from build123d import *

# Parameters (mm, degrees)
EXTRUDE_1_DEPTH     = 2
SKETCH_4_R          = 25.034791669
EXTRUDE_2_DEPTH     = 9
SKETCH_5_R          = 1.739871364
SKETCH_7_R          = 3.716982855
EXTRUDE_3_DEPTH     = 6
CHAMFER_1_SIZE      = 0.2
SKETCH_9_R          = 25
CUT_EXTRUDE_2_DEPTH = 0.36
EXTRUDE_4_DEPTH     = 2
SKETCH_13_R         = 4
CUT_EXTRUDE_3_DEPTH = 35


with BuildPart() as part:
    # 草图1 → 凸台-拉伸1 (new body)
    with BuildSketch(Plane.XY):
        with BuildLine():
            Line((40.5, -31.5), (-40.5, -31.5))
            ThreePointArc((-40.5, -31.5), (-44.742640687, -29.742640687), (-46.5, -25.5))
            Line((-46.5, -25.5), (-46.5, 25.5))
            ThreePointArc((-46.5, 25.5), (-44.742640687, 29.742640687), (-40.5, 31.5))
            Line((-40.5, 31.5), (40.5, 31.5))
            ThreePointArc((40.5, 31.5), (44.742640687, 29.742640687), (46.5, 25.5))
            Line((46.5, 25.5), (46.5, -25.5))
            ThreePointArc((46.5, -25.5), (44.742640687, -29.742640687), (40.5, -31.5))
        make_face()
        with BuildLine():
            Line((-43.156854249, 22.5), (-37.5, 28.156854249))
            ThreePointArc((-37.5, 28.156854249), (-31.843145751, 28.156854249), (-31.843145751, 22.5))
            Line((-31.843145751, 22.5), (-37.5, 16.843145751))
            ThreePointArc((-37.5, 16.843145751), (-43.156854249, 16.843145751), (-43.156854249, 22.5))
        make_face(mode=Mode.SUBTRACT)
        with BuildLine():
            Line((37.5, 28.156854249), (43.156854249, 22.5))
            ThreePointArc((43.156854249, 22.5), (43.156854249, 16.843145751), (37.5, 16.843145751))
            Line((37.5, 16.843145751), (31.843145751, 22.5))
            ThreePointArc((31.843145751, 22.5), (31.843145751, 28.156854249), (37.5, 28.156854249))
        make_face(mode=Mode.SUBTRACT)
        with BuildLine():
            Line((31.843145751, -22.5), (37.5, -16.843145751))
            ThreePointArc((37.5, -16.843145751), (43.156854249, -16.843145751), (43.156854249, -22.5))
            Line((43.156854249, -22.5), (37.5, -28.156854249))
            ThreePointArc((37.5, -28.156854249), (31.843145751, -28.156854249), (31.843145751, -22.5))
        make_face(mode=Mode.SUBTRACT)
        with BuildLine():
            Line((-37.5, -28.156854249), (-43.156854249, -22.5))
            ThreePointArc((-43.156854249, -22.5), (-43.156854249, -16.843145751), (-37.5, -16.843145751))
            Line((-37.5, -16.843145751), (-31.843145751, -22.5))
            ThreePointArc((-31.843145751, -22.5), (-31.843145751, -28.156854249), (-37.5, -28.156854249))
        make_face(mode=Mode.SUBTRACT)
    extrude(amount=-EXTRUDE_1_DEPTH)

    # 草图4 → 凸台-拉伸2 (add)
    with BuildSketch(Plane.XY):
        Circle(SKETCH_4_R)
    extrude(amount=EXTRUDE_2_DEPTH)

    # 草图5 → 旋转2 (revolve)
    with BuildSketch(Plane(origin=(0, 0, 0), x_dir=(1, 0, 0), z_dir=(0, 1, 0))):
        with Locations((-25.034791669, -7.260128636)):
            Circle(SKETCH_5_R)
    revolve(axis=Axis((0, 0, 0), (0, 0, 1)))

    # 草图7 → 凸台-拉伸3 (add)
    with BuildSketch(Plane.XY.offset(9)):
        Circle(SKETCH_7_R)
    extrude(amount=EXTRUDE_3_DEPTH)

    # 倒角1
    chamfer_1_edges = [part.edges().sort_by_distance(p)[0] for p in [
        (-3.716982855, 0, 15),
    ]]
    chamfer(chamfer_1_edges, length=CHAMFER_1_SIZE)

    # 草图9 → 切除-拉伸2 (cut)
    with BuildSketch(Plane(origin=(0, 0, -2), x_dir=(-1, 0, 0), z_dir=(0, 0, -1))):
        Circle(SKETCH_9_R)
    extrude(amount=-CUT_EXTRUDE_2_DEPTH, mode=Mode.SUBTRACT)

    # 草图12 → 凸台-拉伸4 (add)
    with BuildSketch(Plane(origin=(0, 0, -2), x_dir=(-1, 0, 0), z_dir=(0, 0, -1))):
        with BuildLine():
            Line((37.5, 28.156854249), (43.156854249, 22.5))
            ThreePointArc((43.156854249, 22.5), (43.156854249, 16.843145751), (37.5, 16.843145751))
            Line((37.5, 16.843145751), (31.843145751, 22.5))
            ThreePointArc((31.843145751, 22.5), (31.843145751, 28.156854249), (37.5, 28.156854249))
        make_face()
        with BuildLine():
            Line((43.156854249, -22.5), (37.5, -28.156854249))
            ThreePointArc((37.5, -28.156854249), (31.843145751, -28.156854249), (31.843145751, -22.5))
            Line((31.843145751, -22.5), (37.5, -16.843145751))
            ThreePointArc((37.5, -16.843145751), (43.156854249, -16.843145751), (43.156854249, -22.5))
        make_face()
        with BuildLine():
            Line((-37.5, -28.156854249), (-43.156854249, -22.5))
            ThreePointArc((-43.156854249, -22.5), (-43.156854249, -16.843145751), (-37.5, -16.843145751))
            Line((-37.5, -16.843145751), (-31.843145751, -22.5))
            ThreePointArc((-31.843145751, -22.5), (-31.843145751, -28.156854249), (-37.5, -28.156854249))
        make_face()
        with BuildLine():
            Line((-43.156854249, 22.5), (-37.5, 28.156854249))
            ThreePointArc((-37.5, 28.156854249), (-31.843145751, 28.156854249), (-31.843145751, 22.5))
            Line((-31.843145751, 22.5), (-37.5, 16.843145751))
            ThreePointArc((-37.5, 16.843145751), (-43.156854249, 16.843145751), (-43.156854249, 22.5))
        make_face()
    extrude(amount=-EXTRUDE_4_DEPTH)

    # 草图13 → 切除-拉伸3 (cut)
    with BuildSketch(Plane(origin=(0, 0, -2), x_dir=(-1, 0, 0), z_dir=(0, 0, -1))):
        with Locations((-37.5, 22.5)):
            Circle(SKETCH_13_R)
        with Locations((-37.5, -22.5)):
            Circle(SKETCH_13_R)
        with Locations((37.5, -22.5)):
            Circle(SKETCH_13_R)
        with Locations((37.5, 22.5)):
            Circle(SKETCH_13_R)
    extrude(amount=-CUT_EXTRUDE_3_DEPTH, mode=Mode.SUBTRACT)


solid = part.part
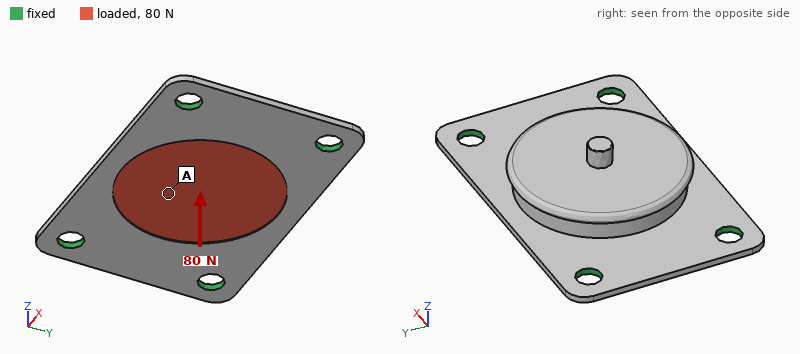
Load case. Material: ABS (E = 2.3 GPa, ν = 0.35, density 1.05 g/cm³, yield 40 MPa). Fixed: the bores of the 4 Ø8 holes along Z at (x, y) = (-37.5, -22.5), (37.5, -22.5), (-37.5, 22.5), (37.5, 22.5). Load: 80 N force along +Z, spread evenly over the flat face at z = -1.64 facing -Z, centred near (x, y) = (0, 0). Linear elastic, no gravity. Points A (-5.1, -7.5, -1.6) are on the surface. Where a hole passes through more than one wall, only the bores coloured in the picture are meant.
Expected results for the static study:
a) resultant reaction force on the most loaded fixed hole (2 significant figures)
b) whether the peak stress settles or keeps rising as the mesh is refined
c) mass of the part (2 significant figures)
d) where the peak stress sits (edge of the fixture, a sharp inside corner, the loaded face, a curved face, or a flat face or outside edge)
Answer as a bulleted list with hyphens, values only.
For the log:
- 28 N
- keeps rising
- 31 g
- edge of the fixture
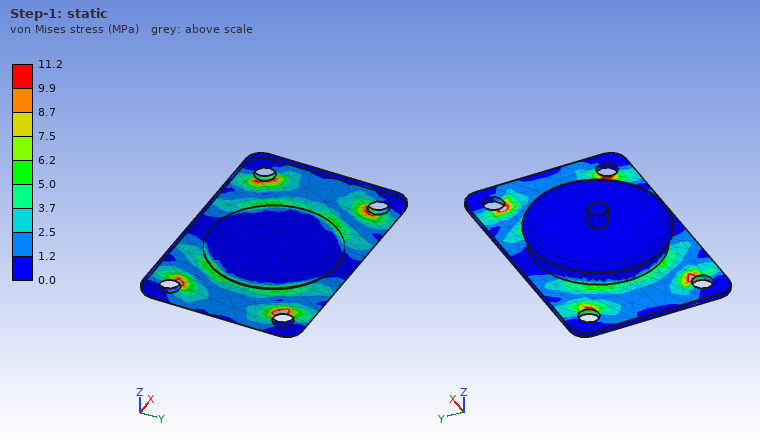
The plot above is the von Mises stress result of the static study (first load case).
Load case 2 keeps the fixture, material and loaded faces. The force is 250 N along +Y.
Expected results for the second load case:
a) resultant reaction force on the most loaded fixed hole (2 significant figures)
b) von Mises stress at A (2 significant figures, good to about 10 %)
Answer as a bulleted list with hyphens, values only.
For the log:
- 70 N
- 0.36 MPa
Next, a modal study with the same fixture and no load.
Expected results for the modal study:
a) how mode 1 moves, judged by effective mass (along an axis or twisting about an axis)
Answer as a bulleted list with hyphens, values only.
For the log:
- along Z
